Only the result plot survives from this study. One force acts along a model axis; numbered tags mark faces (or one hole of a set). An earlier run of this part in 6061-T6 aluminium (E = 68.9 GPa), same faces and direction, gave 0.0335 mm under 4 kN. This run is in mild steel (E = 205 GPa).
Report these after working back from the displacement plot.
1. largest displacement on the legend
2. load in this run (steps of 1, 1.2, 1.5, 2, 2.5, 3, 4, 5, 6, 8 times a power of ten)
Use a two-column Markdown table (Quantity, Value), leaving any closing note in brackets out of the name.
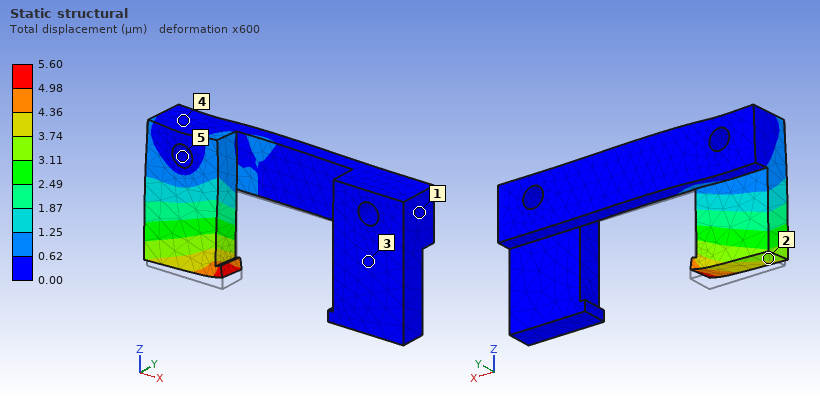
| Quantity | Value |
|---|---|
| largest displacement on the legend | 5.60 µm |
| load in this run | 2 kN |
